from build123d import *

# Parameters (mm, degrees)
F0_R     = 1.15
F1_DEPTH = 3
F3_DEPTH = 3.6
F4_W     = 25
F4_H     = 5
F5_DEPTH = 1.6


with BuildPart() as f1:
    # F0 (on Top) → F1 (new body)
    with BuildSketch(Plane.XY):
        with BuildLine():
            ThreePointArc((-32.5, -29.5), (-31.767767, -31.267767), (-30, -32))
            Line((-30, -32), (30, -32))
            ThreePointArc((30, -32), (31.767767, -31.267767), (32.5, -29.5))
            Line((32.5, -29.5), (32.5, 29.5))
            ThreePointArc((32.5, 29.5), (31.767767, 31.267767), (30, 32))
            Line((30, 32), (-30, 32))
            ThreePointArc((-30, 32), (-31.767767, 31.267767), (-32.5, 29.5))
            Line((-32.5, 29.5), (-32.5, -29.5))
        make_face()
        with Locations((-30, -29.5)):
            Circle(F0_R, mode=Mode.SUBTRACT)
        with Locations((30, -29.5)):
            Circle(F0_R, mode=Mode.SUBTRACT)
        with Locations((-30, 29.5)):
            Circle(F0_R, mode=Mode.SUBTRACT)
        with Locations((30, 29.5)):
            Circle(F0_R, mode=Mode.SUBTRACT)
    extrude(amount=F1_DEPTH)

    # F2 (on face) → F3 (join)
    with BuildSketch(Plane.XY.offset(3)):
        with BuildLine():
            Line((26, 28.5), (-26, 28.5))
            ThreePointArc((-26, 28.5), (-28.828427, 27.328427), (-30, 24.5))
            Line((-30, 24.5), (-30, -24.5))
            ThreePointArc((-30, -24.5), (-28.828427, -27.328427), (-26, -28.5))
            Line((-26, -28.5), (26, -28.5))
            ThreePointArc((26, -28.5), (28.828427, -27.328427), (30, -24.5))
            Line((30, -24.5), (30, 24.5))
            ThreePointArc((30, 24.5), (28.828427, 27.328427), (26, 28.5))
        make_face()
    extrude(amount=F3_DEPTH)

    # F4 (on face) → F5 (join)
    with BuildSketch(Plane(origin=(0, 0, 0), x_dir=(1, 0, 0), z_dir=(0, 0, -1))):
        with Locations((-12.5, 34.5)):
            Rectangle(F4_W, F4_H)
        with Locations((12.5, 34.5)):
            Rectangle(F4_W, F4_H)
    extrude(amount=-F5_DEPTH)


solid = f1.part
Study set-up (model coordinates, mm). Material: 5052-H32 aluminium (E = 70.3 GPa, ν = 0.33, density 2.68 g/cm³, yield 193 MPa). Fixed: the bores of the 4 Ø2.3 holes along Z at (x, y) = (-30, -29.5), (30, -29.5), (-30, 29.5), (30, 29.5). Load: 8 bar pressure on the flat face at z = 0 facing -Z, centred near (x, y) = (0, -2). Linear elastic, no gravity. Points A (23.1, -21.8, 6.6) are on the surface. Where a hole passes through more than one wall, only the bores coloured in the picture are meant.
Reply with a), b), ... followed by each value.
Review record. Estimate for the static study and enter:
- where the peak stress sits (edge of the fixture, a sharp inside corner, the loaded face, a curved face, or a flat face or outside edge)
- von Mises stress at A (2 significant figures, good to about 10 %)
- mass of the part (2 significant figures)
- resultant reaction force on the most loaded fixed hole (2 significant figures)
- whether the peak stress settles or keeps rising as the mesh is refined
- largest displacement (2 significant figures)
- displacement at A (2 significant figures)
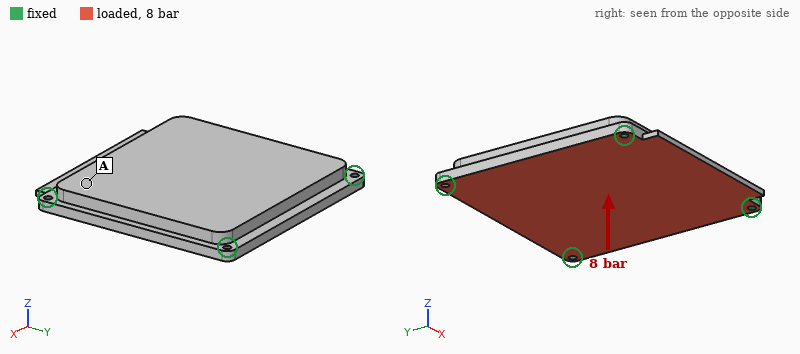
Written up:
a) edge of the fixture
b) 46 MPa
c) 67 g
d) 1.5 kN
e) keeps rising
f) 96 µm
g) 45 µm
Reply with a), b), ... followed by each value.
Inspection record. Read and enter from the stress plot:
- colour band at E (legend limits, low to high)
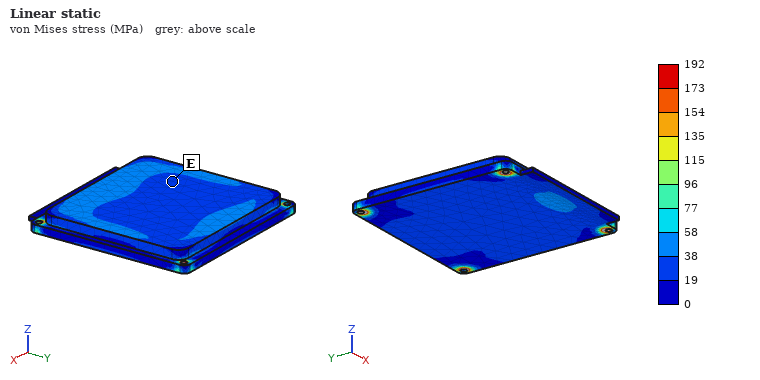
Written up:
a) 19 to 38 MPa
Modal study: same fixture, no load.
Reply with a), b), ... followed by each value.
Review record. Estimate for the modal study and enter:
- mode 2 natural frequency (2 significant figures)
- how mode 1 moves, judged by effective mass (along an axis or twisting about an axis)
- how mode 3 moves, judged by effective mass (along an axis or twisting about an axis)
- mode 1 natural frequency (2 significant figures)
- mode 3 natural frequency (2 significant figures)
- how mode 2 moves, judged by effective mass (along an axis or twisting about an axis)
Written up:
a) 7000 Hz
b) along Z
c) twisting about Y
d) 4100 Hz
e) 7500 Hz
f) twisting about X
